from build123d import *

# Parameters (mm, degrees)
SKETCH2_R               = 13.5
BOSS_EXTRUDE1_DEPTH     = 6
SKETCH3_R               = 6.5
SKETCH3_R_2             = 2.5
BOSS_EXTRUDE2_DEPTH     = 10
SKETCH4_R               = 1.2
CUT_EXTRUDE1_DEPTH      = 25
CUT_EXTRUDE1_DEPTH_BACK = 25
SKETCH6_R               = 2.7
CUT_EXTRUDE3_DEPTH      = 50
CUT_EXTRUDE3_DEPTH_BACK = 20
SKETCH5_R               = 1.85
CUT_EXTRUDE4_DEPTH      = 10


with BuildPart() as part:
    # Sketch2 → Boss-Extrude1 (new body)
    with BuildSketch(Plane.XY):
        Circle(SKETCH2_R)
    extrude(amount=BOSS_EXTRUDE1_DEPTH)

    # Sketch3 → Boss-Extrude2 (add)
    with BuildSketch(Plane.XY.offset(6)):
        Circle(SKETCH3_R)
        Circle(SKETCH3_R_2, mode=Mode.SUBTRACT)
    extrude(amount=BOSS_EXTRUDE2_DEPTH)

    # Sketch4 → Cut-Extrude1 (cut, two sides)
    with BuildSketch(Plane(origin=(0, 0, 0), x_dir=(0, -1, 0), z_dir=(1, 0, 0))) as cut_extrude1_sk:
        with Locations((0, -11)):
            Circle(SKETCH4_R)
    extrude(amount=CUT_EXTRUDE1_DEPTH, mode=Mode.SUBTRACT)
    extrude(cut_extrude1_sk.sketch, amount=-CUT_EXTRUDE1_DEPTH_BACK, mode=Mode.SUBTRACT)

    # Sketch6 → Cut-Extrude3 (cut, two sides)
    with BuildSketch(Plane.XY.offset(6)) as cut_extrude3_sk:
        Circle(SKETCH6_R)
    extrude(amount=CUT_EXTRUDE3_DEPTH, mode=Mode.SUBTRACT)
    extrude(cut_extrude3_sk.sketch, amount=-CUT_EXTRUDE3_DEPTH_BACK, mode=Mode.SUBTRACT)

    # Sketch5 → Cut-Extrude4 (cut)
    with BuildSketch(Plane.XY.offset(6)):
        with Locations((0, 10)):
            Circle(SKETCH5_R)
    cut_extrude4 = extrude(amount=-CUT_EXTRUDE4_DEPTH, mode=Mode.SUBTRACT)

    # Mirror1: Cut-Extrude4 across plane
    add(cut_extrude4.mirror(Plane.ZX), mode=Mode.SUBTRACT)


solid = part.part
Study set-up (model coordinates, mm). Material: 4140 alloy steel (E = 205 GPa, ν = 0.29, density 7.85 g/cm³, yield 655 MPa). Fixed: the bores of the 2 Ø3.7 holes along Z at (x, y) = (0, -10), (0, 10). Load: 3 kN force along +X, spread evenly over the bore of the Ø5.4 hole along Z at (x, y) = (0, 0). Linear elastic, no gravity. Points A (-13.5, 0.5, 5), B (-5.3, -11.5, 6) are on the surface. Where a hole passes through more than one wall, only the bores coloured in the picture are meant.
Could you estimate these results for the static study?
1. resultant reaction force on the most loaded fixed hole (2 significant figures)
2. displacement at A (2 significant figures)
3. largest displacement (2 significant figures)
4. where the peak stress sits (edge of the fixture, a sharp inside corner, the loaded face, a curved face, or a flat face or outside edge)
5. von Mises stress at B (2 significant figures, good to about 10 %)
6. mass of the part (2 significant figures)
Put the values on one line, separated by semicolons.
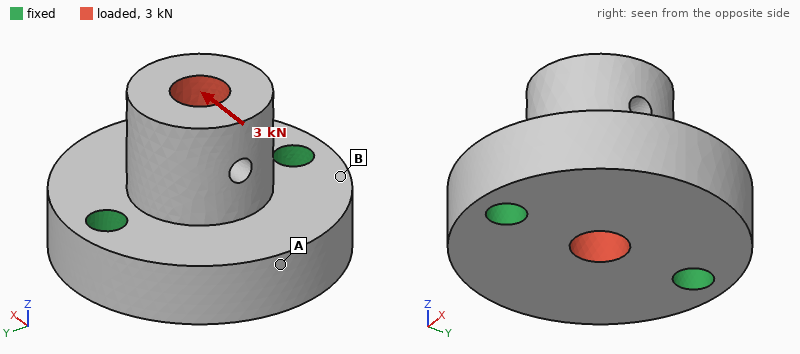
1.5 kN; 6.9 µm; 12 µm; edge of the fixture; 34 MPa; 33 g
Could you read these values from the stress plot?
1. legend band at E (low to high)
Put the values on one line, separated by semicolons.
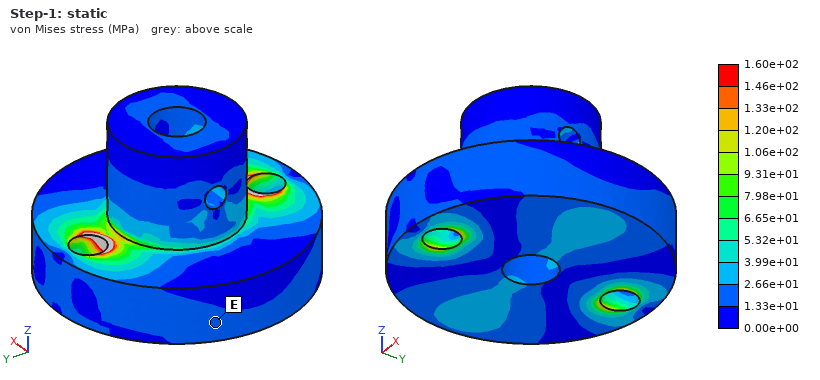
1.33e+01 to 2.66e+01 MPa
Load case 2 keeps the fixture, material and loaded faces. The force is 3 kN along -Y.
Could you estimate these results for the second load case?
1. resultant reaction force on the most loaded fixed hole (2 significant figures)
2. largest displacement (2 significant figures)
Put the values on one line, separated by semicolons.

1.7 kN; 5.5 µm
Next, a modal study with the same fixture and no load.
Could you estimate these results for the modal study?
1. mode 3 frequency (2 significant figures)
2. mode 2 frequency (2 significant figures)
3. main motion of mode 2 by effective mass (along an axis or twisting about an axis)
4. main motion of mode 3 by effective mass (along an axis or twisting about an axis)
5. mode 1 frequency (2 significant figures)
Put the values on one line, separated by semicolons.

37 kHz; 31 kHz; along Z; along Y; 19 kHz
